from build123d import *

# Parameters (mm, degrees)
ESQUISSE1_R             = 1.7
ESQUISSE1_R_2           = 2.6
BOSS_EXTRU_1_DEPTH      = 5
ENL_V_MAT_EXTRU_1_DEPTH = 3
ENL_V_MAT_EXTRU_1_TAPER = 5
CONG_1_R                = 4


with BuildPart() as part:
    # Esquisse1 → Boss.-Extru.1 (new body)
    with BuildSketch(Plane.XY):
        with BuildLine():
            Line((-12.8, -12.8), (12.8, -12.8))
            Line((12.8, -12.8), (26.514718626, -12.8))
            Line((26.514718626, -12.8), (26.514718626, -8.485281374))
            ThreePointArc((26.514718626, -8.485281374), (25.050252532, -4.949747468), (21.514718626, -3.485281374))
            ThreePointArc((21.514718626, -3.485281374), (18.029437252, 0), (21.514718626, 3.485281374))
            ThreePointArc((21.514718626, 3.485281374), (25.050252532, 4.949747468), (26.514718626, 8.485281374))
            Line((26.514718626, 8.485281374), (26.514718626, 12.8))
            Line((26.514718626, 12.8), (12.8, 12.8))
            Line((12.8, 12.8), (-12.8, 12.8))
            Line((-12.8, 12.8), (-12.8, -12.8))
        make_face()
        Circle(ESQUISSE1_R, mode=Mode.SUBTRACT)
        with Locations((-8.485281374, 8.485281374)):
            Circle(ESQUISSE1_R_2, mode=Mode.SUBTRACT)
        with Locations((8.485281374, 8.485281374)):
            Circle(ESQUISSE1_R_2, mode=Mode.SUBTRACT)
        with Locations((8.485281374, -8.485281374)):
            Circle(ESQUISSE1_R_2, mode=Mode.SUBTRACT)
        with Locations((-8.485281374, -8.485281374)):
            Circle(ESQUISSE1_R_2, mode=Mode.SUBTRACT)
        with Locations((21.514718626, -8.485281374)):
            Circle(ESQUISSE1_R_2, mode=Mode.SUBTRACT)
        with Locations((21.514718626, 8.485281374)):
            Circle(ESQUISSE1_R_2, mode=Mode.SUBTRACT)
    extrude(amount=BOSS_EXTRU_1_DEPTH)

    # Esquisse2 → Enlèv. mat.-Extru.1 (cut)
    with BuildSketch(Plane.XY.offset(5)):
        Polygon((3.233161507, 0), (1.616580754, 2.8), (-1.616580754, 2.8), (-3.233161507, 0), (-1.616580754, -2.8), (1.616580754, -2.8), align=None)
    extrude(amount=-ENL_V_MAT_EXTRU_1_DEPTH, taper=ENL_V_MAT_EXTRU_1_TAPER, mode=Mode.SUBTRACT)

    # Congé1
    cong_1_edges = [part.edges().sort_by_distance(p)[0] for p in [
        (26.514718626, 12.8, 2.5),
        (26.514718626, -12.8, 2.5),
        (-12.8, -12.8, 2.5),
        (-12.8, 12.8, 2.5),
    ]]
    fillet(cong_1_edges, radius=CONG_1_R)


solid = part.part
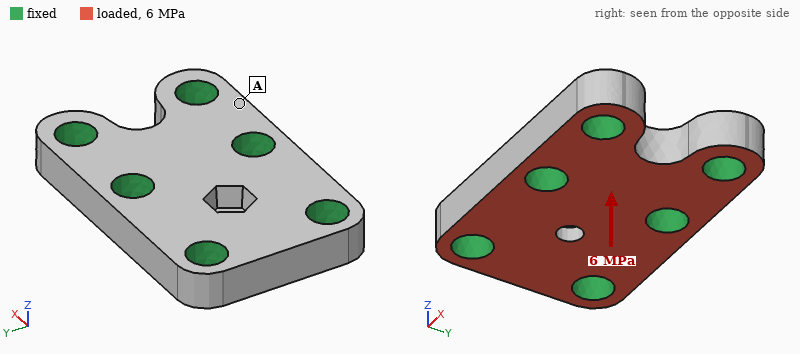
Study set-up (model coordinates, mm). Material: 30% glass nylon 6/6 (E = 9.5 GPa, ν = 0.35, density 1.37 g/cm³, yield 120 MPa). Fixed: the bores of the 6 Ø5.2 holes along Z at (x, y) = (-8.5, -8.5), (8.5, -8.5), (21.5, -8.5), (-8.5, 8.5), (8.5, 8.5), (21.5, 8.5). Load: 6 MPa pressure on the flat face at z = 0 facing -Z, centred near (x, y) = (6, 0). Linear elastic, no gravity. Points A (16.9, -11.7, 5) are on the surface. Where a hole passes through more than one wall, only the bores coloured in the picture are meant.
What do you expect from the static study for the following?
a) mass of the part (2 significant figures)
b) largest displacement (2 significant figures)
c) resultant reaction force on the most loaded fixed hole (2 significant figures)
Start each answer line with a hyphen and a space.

- 5.4 g
- 30 µm
- 1.0 kN
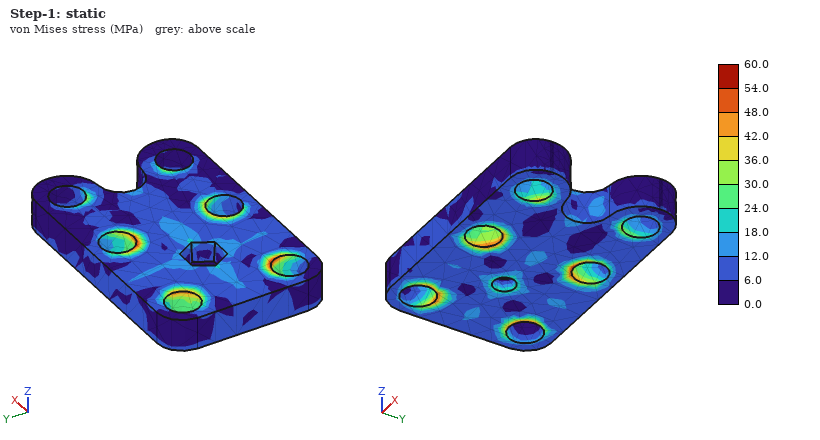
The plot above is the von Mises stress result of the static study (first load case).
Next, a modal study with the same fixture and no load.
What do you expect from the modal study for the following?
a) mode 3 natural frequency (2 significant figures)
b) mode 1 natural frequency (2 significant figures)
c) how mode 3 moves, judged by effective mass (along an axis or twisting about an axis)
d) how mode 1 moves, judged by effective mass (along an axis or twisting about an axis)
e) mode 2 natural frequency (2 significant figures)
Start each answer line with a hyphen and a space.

- 47 kHz
- 36 kHz
- twisting about X
- along Z
- 43 kHz
